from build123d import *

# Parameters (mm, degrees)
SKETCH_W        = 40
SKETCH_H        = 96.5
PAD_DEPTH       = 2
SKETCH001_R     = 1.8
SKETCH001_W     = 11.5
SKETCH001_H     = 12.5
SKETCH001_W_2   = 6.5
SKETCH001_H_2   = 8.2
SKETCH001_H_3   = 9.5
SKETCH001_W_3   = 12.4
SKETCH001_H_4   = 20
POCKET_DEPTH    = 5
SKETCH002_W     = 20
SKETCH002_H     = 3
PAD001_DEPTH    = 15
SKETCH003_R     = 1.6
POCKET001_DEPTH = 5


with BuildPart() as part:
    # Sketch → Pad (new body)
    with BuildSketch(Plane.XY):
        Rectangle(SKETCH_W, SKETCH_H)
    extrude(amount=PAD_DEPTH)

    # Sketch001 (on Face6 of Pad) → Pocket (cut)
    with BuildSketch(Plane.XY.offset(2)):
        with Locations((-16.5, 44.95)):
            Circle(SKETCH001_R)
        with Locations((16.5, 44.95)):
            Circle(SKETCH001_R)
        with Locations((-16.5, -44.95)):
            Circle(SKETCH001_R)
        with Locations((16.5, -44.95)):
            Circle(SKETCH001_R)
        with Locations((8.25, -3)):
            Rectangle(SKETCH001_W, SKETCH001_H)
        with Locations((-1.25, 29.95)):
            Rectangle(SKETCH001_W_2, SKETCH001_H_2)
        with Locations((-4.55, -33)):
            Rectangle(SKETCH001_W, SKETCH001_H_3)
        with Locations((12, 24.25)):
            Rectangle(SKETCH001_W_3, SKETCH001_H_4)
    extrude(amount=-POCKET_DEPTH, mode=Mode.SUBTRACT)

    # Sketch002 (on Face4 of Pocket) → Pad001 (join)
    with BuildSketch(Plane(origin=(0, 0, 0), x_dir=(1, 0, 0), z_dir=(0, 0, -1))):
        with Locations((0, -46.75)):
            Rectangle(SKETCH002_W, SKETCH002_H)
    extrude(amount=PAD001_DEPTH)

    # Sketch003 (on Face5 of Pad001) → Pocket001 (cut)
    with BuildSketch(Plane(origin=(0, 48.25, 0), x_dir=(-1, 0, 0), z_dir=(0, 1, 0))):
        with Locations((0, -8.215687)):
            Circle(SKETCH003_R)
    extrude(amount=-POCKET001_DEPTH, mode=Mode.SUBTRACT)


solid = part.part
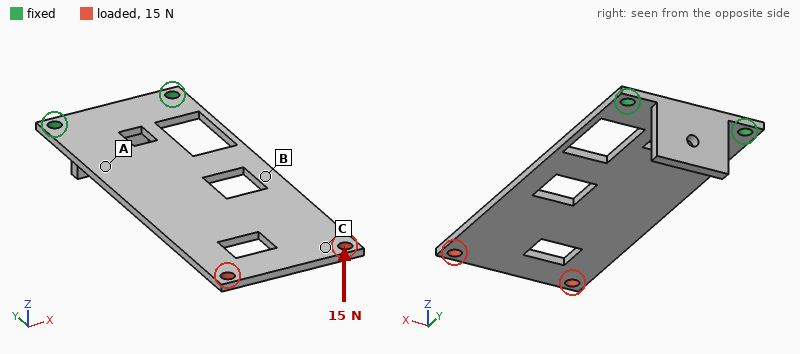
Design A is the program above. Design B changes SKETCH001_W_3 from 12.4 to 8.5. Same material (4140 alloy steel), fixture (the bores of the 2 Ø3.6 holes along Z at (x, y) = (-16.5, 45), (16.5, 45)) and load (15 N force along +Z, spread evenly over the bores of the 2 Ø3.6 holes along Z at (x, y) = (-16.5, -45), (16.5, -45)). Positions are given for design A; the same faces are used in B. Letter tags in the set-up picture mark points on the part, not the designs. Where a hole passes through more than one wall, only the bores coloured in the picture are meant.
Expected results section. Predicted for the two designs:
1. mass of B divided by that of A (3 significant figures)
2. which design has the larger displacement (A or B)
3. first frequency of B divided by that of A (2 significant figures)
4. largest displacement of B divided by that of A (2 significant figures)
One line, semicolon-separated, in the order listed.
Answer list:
1.02; A; 1.1; 0.89
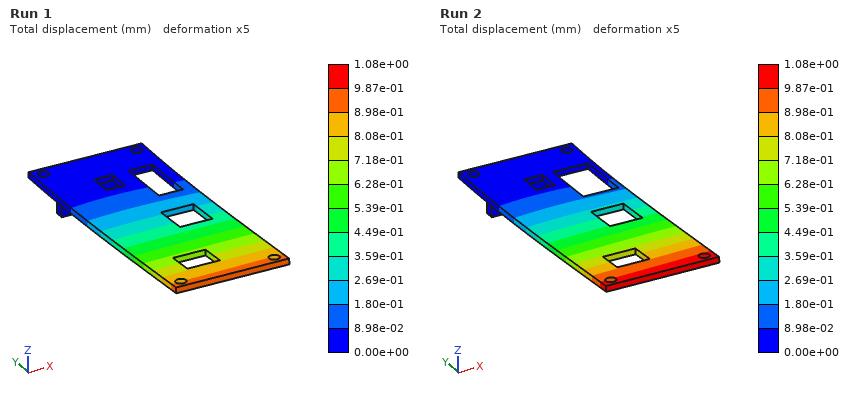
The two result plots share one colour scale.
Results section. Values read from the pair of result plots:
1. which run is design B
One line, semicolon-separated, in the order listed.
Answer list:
Run 1
